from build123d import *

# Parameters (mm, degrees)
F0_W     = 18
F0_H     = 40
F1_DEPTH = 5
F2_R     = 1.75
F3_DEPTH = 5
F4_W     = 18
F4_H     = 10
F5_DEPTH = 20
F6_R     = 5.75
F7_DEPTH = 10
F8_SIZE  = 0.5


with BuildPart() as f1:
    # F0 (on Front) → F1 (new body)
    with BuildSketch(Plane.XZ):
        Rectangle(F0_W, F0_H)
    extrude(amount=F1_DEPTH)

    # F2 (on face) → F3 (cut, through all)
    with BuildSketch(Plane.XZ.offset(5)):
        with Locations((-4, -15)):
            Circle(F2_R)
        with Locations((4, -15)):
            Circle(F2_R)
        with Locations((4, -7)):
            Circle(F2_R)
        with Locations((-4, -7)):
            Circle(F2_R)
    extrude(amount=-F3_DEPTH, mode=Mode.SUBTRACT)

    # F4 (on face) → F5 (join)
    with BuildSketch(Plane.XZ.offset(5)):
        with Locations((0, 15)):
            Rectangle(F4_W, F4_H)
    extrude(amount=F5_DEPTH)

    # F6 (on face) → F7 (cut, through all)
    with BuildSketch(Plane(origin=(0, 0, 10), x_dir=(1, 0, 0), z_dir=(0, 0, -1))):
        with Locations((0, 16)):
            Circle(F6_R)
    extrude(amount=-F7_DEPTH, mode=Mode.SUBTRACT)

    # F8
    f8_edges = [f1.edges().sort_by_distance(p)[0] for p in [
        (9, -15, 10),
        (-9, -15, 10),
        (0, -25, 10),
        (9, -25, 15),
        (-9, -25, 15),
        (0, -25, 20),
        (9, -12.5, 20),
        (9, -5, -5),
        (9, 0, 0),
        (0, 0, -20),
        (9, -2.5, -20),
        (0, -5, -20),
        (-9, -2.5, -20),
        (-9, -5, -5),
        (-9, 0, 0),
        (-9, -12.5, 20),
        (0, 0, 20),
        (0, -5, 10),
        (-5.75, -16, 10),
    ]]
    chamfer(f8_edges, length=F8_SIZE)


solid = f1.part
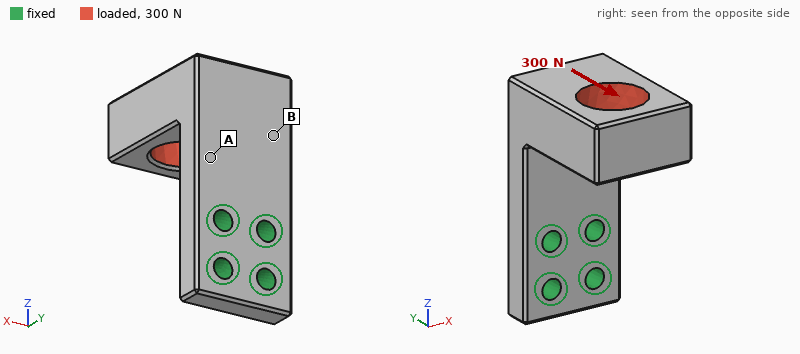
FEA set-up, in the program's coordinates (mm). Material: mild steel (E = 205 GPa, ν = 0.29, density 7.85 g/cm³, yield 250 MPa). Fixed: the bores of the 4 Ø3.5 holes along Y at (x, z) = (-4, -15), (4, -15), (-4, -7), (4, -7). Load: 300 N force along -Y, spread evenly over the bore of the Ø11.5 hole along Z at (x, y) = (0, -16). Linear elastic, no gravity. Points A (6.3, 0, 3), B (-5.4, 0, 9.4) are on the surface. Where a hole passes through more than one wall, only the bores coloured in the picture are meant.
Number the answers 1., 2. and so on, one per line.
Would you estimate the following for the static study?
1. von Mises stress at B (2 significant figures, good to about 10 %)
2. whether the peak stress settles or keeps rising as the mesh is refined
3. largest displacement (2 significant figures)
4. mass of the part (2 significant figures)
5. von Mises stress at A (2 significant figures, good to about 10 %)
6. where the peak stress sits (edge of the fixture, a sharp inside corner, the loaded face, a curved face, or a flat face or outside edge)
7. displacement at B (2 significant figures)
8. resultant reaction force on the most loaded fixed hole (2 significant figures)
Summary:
1. 22 MPa
2. keeps rising
3. 52 µm
4. 47 g
5. 49 MPa
6. edge of the fixture
7. 17 µm
8. 200 N
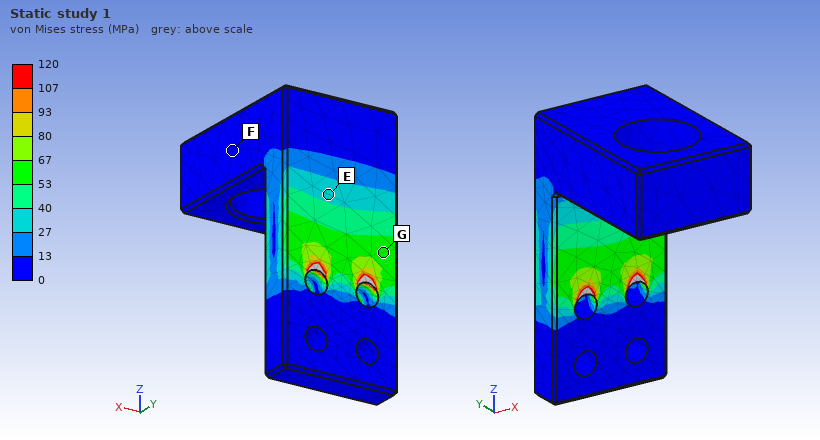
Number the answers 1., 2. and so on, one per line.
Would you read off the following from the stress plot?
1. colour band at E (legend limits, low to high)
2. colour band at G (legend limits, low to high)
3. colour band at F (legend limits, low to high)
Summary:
1. 27 to 40 MPa
2. 53 to 67 MPa
3. 0 to 13 MPa
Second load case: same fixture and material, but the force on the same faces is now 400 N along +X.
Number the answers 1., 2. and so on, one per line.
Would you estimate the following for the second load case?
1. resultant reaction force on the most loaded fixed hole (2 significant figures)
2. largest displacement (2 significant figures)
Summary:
1. 820 N
2. 40 µm
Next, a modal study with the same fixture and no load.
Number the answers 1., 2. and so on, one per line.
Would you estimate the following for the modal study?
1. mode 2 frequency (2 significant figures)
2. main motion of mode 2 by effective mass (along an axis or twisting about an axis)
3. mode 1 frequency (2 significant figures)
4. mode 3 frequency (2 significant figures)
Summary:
1. 4200 Hz
2. along X
3. 2500 Hz
4. 9400 Hz
